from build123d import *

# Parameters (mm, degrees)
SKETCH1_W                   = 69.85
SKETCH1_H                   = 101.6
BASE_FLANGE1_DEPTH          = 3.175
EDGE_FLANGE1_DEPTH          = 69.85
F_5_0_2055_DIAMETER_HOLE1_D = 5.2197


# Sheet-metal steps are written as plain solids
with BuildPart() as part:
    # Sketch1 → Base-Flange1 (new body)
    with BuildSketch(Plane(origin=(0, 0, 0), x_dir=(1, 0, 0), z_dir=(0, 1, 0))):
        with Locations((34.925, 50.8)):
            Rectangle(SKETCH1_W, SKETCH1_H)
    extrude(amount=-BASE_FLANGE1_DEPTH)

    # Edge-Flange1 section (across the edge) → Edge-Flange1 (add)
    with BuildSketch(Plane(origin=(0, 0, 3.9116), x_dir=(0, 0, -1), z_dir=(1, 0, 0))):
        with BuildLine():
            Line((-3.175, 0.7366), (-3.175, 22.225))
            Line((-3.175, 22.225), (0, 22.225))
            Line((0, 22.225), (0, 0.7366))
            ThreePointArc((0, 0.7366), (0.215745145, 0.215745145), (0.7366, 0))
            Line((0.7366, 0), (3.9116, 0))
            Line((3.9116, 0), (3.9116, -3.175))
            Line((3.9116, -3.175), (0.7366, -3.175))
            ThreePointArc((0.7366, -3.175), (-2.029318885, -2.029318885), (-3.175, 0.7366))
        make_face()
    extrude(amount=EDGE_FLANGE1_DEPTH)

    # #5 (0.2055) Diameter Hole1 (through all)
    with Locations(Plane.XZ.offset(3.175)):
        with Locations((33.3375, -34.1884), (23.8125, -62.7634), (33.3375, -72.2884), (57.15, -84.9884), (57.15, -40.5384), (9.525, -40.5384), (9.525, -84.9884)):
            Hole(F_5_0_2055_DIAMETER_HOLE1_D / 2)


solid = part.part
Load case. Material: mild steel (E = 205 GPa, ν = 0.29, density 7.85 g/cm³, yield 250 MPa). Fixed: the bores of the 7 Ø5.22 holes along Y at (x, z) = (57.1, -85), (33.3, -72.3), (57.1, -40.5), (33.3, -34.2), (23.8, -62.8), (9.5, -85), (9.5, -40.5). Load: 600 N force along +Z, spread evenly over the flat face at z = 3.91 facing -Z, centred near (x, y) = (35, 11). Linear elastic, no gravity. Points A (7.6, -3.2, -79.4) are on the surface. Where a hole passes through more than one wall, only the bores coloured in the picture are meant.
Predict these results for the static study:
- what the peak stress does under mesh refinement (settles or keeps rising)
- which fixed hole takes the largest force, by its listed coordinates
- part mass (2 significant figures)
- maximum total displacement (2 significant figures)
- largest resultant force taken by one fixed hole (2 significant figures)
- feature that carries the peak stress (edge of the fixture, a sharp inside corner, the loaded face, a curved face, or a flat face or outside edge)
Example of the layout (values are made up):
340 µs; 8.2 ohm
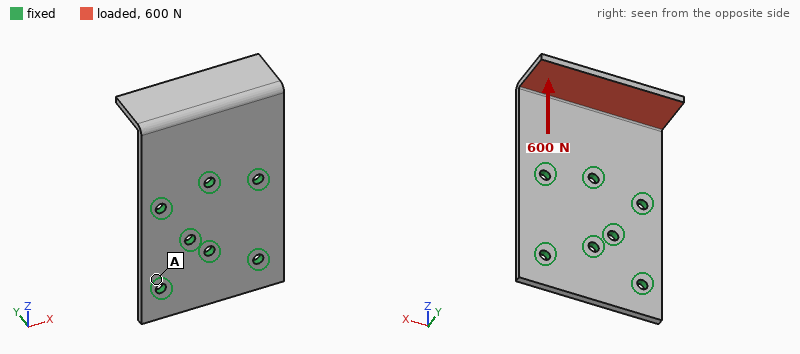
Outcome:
keeps rising; (33.3, -34.2); 220 g; 0.28 mm; 260 N; edge of the fixture
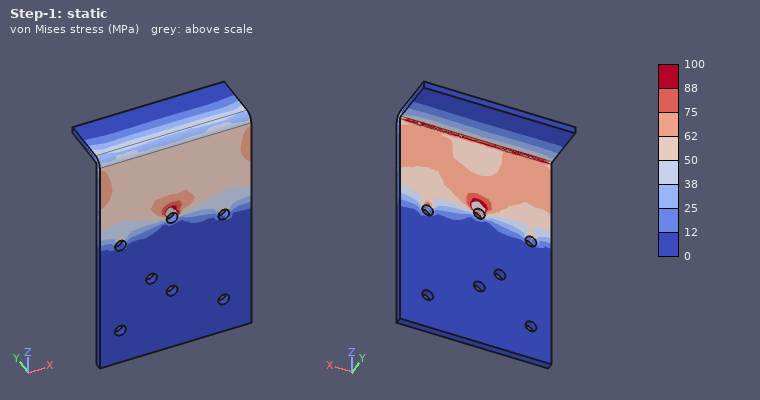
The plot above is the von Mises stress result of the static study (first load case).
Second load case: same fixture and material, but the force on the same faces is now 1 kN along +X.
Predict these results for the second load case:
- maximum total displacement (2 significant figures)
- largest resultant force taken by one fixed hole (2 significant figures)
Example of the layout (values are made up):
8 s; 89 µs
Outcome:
0.24 mm; 750 N
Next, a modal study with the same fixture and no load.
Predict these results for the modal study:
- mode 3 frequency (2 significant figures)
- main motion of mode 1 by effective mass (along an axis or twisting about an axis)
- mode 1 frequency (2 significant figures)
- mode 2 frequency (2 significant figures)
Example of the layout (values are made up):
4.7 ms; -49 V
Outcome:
2900 Hz; along Y; 780 Hz; 1400 Hz
